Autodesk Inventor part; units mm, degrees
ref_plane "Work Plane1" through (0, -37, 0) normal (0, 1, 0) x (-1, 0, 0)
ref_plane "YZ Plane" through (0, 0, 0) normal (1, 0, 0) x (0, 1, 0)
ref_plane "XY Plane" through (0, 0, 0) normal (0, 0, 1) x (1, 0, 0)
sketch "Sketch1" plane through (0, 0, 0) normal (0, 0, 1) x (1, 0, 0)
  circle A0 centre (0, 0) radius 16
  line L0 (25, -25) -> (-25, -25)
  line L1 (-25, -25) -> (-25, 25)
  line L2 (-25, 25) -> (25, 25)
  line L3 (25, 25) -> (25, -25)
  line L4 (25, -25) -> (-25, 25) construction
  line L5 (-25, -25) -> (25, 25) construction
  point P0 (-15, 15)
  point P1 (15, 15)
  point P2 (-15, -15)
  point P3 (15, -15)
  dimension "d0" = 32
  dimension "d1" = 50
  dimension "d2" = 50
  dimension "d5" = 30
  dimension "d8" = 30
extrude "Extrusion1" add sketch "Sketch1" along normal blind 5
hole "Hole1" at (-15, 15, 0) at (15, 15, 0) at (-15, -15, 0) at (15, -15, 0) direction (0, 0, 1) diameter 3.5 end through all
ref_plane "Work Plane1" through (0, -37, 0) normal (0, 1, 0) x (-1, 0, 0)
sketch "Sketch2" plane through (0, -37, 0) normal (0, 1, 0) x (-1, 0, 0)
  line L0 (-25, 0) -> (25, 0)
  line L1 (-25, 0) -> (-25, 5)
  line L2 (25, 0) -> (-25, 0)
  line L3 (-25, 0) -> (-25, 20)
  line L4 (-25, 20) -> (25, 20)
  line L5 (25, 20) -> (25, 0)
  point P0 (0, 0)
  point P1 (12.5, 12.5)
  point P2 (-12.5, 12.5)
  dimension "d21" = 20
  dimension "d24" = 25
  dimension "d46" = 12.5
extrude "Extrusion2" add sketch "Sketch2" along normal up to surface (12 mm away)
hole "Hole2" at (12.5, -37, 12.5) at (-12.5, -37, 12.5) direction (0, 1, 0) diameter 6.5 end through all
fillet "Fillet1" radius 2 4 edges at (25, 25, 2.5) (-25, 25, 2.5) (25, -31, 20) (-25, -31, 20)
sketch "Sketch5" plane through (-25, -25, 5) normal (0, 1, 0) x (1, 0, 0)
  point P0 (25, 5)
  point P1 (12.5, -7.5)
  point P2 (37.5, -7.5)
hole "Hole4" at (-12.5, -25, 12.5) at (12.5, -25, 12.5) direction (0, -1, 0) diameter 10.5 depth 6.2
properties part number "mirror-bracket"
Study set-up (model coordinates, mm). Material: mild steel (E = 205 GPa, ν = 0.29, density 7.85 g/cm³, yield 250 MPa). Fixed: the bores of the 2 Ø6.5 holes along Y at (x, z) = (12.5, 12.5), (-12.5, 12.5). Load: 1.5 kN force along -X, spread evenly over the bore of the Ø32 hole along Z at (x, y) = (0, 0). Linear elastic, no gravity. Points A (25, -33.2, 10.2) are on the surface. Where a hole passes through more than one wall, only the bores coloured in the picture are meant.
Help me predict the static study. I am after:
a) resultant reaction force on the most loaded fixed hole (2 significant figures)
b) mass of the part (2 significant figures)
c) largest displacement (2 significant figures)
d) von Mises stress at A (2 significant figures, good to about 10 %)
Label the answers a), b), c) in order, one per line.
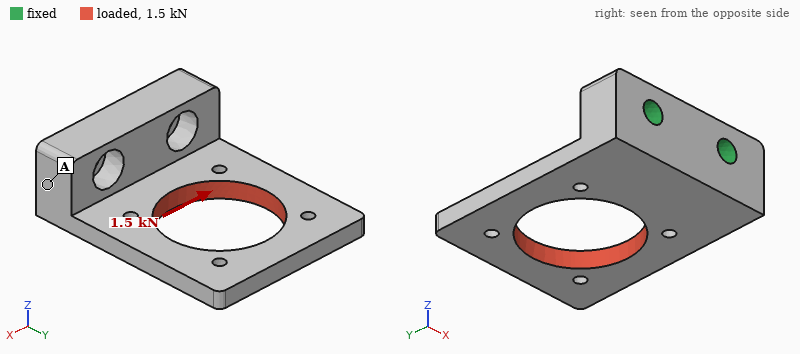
a) 1.9 kN
b) 150 g
c) 33 µm
d) 11 MPa
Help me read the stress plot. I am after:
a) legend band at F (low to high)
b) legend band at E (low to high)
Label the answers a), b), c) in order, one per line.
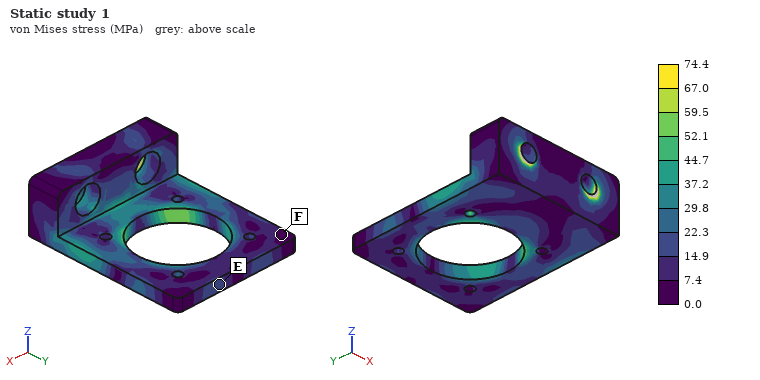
a) 0.0 to 7.4 MPa
b) 14.9 to 22.3 MPa
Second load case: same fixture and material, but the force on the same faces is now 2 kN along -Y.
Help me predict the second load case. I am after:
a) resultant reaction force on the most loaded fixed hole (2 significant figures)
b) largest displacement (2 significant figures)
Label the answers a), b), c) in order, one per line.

a) 1.0 kN
b) 20 µm
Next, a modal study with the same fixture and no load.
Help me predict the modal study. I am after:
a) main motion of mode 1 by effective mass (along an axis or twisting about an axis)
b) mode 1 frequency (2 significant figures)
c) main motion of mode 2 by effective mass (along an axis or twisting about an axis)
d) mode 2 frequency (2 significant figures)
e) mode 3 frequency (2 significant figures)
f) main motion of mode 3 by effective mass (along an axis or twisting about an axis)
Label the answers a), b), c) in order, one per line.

a) along Z
b) 1200 Hz
c) twisting about Y
d) 2900 Hz
e) 4800 Hz
f) along X
